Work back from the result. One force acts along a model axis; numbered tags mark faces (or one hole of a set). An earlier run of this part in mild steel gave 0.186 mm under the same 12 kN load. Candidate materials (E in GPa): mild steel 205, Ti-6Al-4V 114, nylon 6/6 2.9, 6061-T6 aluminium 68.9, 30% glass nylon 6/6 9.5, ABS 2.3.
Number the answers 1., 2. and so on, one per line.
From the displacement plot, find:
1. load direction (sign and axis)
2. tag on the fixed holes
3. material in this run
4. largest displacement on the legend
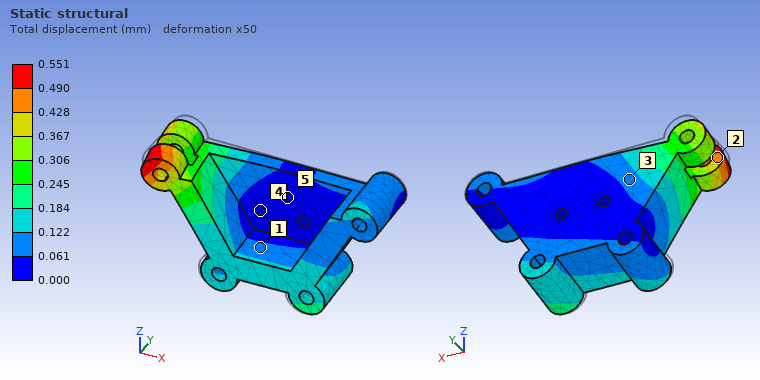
1. -Y
2. 4
3. 6061-T6 aluminium
4. 0.551 mm
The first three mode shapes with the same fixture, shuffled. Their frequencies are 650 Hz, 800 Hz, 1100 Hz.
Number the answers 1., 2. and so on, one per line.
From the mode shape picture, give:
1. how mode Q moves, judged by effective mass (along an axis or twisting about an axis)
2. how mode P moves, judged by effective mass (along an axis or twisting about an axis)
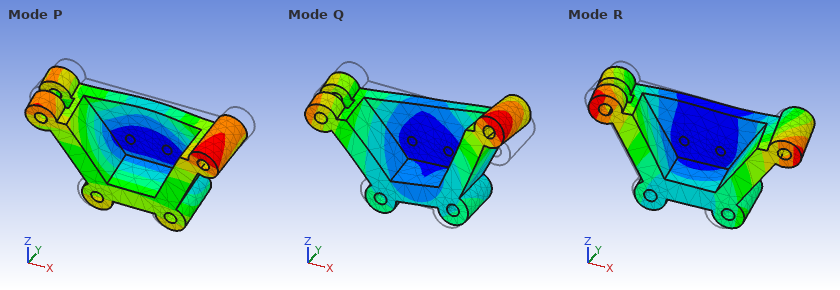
1. twisting about Y
2. along Z
